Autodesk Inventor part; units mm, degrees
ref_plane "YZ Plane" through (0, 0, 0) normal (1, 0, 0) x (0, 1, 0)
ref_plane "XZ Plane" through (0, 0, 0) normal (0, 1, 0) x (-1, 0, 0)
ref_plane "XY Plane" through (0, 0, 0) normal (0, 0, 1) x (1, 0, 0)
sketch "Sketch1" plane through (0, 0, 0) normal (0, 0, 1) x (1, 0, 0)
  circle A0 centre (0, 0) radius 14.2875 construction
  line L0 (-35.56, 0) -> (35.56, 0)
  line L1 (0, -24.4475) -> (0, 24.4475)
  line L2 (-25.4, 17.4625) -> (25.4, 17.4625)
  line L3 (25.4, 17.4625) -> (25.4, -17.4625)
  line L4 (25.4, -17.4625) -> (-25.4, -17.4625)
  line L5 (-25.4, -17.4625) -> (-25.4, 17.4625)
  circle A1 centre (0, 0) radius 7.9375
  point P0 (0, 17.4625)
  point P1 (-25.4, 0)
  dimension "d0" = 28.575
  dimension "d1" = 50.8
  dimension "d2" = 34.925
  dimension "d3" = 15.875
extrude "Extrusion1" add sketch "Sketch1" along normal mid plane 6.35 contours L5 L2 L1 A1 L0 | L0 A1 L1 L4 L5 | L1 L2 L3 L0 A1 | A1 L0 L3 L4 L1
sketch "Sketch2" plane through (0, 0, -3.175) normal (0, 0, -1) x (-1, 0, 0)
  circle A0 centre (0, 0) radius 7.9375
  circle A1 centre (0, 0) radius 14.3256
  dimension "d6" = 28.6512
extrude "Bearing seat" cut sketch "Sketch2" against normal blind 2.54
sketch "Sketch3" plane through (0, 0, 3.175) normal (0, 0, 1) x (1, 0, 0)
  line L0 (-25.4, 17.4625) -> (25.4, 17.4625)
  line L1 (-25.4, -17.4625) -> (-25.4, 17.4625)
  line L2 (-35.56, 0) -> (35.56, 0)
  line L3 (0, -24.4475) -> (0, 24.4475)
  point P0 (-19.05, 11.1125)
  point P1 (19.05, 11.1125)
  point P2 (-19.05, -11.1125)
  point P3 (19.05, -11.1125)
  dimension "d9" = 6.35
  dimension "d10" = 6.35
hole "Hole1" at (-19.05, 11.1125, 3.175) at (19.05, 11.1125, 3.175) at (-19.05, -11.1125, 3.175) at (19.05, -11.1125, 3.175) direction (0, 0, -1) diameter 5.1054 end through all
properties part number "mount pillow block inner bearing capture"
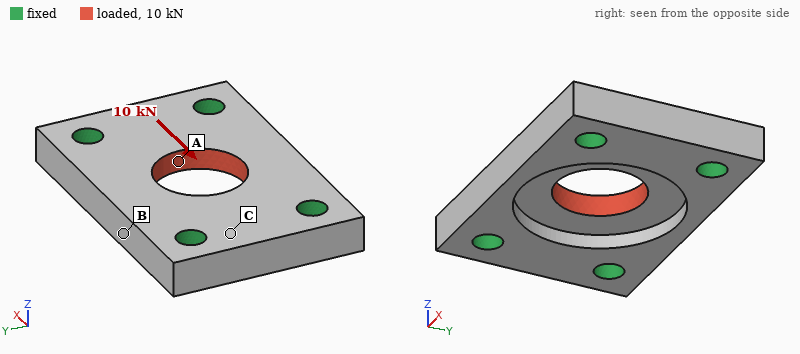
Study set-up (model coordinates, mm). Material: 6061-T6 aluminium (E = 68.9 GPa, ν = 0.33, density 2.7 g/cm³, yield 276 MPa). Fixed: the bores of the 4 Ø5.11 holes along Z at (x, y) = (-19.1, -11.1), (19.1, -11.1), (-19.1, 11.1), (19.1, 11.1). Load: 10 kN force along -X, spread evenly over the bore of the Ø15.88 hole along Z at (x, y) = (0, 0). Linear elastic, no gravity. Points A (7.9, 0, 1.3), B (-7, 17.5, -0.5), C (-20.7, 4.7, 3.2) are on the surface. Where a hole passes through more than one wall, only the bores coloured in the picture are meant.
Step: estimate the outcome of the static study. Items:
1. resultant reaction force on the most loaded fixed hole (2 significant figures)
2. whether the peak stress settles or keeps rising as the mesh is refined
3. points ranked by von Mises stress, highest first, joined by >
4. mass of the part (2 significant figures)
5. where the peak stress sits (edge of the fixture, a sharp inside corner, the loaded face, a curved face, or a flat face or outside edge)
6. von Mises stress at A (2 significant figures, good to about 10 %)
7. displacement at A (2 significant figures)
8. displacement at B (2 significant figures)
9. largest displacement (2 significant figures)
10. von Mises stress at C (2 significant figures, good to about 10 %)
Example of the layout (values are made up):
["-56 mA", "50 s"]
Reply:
["2.6 kN", "keeps rising", "A > C > B", "23 g", "edge of the fixture", "45 MPa", "11 µm", "3.0 µm", "12 µm", "25 MPa"]
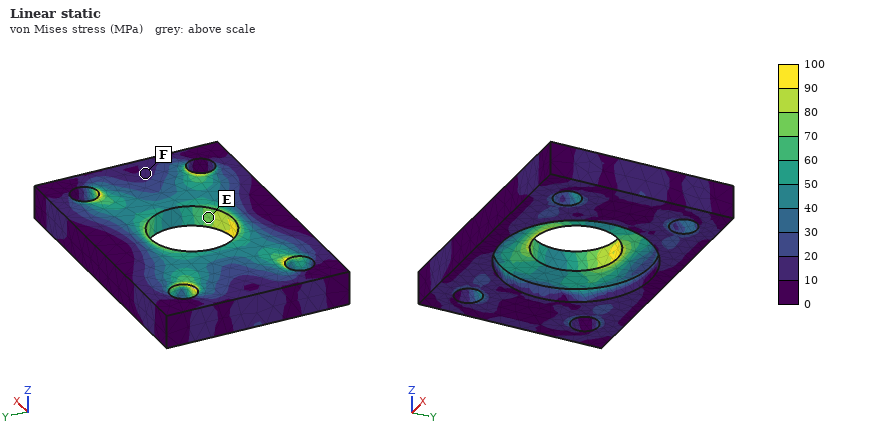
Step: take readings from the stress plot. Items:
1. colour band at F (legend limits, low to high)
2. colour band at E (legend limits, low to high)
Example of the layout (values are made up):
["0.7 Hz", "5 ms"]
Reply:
["10 to 20 MPa", "70 to 80 MPa"]
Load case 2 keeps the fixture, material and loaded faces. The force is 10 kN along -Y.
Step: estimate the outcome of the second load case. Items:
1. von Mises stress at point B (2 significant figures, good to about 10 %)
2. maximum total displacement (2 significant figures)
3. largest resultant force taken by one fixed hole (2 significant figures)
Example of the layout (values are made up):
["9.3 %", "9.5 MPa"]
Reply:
["27 MPa", "28 µm", "2.8 kN"]
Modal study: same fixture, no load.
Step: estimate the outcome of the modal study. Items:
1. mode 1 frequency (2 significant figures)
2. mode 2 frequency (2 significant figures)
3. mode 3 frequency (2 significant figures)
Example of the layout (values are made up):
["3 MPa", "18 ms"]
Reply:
["23 kHz", "24 kHz", "35 kHz"]
